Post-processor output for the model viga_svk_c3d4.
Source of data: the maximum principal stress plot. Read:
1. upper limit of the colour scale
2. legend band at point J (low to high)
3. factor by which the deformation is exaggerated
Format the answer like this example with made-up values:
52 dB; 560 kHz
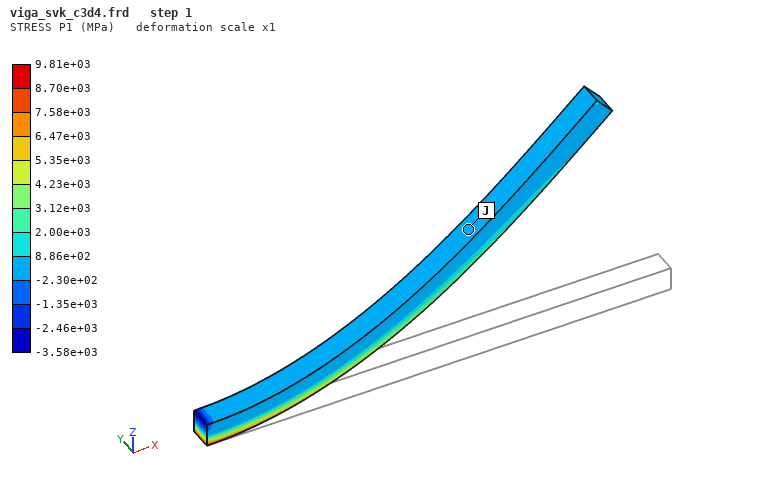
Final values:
9.81e+03 MPa; -2.30e+02 to 8.86e+02 MPa; 1
